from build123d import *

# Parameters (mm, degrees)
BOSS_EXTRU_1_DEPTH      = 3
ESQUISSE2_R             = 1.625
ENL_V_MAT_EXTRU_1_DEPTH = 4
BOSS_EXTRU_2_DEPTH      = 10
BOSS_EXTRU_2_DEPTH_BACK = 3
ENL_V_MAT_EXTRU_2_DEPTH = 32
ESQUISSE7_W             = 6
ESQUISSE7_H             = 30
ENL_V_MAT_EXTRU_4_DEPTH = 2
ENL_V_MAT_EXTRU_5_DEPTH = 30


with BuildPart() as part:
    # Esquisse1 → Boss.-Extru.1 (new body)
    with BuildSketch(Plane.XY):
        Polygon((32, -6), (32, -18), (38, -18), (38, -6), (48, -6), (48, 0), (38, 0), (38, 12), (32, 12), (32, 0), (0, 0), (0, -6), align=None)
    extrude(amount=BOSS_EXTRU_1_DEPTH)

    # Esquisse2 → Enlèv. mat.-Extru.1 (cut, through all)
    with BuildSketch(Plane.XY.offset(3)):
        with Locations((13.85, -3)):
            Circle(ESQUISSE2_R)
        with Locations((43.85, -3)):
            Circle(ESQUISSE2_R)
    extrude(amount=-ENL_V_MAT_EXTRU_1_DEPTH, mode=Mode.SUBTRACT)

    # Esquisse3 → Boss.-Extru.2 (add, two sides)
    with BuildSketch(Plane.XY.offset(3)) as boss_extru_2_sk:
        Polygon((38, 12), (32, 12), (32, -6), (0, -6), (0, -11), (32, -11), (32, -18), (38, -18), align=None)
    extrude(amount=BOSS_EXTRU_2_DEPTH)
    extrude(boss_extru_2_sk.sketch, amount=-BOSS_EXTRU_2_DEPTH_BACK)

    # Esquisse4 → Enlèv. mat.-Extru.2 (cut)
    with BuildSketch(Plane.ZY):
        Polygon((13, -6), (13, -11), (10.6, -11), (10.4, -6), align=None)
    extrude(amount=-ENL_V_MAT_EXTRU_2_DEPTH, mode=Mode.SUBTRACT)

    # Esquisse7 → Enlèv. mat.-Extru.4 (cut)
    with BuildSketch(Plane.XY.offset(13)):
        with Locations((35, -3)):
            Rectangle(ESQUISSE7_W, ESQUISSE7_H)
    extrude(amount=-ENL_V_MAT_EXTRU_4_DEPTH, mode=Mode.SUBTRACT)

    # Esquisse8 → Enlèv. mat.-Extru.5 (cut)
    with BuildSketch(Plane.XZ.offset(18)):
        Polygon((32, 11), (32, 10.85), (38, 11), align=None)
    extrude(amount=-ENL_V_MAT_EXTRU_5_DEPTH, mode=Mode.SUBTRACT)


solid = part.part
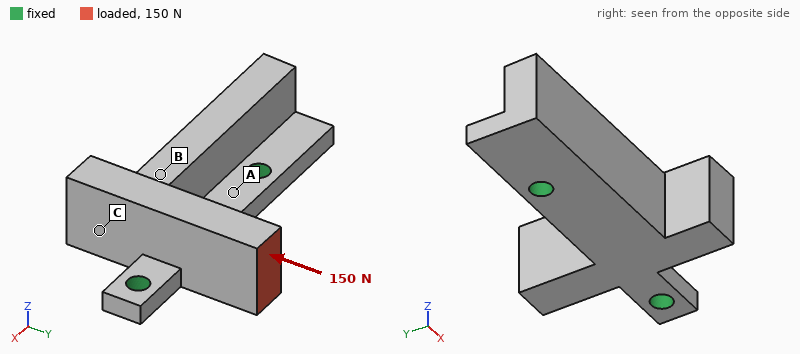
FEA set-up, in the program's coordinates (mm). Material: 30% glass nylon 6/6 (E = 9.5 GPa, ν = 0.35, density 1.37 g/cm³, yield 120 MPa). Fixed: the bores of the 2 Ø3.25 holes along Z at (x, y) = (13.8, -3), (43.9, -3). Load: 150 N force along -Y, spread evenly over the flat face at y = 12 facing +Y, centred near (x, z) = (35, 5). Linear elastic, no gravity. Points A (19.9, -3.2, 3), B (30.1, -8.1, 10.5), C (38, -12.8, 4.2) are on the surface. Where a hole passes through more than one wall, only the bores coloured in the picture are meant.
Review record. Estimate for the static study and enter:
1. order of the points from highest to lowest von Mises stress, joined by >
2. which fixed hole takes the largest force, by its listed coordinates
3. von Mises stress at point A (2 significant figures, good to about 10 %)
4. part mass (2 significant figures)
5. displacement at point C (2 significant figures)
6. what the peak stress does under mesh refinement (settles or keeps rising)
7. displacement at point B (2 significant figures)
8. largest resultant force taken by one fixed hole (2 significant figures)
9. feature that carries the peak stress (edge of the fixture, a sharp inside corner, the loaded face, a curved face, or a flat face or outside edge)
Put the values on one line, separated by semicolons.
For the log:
A > B > C; (43.9, -3); 11 MPa; 6.0 g; 0.085 mm; keeps rising; 0.088 mm; 110 N; edge of the fixture
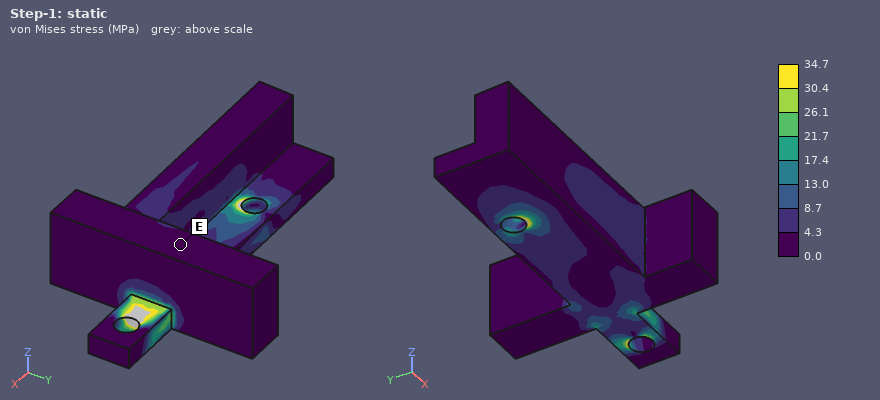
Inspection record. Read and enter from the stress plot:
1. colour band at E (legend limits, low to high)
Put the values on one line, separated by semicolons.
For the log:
0.0 to 4.3 MPa
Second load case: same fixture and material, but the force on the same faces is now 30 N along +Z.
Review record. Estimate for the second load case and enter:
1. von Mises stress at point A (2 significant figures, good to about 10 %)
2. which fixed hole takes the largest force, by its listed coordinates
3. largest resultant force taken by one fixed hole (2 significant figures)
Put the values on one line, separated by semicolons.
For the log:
7.4 MPa; (43.9, -3); 26 N
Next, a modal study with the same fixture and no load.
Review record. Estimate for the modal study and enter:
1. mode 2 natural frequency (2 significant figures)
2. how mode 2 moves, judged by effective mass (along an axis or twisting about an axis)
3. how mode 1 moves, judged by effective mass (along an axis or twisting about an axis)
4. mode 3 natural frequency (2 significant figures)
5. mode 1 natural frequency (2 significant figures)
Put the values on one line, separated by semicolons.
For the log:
5700 Hz; along Z; along Y; 6500 Hz; 2400 Hz
